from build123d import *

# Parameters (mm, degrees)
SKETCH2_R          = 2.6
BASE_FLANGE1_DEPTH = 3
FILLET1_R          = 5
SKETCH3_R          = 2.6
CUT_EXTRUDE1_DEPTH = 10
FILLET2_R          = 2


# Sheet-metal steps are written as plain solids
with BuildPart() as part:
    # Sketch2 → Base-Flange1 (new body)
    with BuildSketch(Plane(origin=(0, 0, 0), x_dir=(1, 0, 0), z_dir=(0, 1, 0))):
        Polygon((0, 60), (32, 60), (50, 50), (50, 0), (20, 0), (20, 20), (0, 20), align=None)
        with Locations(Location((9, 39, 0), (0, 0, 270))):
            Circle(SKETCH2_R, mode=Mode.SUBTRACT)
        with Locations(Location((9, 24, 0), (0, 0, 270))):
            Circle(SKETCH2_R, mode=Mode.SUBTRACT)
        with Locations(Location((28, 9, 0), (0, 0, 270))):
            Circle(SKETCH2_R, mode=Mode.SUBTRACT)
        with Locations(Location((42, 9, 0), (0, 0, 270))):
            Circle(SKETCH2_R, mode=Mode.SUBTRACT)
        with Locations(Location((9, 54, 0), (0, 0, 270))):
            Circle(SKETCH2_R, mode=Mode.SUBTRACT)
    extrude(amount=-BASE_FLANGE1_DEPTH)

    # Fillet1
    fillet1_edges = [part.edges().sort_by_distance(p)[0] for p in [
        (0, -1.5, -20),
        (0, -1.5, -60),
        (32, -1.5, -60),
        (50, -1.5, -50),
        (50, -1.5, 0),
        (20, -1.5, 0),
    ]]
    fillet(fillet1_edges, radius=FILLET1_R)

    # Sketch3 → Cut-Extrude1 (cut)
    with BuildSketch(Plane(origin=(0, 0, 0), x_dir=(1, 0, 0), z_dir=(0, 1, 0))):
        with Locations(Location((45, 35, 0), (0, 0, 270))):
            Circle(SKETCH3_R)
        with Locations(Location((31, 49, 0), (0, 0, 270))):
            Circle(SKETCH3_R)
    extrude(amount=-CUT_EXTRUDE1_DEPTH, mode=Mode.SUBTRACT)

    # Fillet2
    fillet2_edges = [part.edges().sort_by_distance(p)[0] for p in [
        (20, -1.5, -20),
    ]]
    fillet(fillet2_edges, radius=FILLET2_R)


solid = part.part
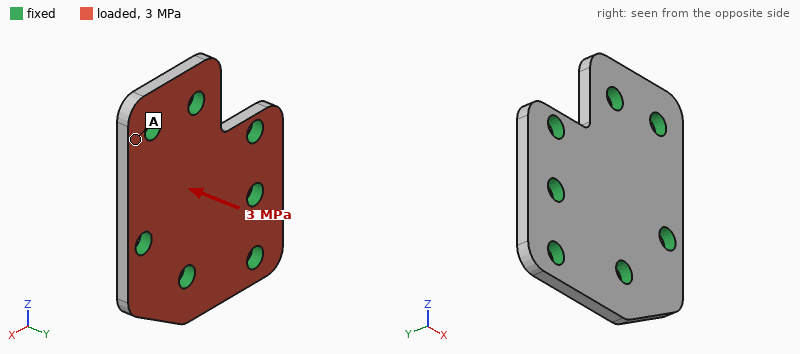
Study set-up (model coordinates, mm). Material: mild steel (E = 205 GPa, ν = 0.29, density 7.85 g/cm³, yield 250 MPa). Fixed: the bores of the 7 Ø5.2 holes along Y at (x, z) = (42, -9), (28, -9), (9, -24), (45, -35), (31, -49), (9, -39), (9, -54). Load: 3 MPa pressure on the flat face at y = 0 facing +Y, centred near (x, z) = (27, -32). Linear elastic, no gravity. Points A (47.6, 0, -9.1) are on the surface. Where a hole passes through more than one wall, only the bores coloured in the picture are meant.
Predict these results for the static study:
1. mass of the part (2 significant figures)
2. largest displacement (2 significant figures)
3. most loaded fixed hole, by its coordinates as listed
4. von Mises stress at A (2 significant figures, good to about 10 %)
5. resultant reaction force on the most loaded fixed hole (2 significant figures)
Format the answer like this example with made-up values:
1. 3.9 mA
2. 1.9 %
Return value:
1. 55 g
2. 15 µm
3. (31, -49)
4. 32 MPa
5. 1.4 kN
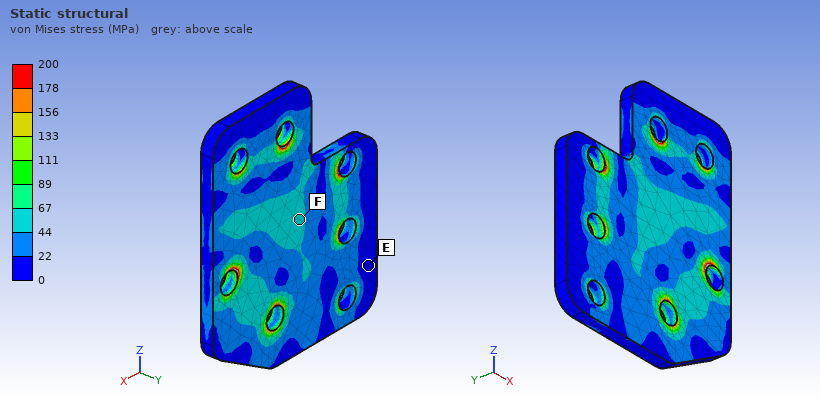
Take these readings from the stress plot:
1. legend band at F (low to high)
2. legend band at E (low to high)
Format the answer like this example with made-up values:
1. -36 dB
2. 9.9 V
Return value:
1. 44 to 67 MPa
2. 0 to 22 MPa
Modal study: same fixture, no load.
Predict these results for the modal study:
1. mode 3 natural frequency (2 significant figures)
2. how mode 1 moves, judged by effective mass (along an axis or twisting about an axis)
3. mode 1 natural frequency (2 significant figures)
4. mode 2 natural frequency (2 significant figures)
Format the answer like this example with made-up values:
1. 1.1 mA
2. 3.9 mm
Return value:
1. 27 kHz
2. along Y
3. 18 kHz
4. 20 kHz
